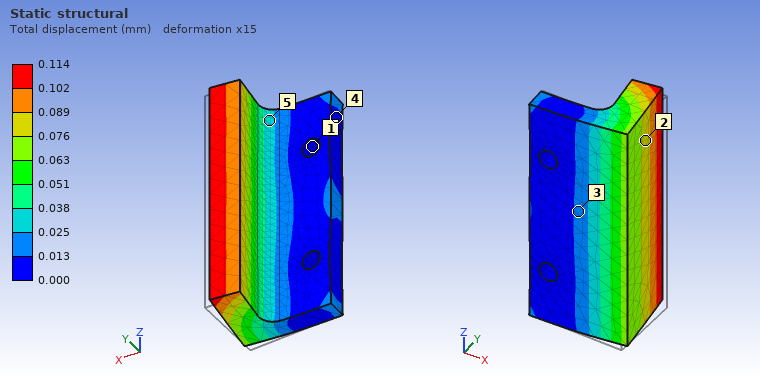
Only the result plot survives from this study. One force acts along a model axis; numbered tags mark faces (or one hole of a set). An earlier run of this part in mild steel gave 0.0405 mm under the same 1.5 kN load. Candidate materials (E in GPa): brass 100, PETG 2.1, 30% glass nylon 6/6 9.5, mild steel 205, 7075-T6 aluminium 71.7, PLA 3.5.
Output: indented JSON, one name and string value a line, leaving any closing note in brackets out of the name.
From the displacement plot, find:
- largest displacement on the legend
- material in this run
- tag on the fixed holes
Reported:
{
  "largest displacement on the legend": "0.114 mm",
  "material in this run": "7075-T6 aluminium",
  "tag on the fixed holes": "1"
}
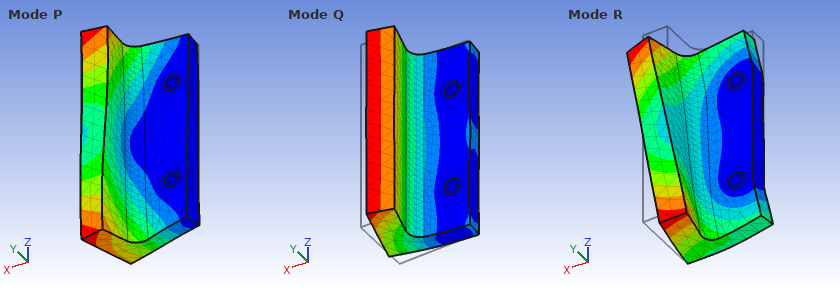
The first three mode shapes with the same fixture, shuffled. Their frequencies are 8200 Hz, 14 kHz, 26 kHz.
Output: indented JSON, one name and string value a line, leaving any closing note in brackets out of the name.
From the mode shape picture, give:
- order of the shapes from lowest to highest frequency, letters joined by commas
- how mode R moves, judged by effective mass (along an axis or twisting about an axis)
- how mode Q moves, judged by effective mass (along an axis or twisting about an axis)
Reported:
{
  "order of the shapes from lowest to highest frequency, letters joined by commas": "Q, P, R",
  "how mode R moves, judged by effective mass": "along Z",
  "how mode Q moves, judged by effective mass": "along Y"
}
